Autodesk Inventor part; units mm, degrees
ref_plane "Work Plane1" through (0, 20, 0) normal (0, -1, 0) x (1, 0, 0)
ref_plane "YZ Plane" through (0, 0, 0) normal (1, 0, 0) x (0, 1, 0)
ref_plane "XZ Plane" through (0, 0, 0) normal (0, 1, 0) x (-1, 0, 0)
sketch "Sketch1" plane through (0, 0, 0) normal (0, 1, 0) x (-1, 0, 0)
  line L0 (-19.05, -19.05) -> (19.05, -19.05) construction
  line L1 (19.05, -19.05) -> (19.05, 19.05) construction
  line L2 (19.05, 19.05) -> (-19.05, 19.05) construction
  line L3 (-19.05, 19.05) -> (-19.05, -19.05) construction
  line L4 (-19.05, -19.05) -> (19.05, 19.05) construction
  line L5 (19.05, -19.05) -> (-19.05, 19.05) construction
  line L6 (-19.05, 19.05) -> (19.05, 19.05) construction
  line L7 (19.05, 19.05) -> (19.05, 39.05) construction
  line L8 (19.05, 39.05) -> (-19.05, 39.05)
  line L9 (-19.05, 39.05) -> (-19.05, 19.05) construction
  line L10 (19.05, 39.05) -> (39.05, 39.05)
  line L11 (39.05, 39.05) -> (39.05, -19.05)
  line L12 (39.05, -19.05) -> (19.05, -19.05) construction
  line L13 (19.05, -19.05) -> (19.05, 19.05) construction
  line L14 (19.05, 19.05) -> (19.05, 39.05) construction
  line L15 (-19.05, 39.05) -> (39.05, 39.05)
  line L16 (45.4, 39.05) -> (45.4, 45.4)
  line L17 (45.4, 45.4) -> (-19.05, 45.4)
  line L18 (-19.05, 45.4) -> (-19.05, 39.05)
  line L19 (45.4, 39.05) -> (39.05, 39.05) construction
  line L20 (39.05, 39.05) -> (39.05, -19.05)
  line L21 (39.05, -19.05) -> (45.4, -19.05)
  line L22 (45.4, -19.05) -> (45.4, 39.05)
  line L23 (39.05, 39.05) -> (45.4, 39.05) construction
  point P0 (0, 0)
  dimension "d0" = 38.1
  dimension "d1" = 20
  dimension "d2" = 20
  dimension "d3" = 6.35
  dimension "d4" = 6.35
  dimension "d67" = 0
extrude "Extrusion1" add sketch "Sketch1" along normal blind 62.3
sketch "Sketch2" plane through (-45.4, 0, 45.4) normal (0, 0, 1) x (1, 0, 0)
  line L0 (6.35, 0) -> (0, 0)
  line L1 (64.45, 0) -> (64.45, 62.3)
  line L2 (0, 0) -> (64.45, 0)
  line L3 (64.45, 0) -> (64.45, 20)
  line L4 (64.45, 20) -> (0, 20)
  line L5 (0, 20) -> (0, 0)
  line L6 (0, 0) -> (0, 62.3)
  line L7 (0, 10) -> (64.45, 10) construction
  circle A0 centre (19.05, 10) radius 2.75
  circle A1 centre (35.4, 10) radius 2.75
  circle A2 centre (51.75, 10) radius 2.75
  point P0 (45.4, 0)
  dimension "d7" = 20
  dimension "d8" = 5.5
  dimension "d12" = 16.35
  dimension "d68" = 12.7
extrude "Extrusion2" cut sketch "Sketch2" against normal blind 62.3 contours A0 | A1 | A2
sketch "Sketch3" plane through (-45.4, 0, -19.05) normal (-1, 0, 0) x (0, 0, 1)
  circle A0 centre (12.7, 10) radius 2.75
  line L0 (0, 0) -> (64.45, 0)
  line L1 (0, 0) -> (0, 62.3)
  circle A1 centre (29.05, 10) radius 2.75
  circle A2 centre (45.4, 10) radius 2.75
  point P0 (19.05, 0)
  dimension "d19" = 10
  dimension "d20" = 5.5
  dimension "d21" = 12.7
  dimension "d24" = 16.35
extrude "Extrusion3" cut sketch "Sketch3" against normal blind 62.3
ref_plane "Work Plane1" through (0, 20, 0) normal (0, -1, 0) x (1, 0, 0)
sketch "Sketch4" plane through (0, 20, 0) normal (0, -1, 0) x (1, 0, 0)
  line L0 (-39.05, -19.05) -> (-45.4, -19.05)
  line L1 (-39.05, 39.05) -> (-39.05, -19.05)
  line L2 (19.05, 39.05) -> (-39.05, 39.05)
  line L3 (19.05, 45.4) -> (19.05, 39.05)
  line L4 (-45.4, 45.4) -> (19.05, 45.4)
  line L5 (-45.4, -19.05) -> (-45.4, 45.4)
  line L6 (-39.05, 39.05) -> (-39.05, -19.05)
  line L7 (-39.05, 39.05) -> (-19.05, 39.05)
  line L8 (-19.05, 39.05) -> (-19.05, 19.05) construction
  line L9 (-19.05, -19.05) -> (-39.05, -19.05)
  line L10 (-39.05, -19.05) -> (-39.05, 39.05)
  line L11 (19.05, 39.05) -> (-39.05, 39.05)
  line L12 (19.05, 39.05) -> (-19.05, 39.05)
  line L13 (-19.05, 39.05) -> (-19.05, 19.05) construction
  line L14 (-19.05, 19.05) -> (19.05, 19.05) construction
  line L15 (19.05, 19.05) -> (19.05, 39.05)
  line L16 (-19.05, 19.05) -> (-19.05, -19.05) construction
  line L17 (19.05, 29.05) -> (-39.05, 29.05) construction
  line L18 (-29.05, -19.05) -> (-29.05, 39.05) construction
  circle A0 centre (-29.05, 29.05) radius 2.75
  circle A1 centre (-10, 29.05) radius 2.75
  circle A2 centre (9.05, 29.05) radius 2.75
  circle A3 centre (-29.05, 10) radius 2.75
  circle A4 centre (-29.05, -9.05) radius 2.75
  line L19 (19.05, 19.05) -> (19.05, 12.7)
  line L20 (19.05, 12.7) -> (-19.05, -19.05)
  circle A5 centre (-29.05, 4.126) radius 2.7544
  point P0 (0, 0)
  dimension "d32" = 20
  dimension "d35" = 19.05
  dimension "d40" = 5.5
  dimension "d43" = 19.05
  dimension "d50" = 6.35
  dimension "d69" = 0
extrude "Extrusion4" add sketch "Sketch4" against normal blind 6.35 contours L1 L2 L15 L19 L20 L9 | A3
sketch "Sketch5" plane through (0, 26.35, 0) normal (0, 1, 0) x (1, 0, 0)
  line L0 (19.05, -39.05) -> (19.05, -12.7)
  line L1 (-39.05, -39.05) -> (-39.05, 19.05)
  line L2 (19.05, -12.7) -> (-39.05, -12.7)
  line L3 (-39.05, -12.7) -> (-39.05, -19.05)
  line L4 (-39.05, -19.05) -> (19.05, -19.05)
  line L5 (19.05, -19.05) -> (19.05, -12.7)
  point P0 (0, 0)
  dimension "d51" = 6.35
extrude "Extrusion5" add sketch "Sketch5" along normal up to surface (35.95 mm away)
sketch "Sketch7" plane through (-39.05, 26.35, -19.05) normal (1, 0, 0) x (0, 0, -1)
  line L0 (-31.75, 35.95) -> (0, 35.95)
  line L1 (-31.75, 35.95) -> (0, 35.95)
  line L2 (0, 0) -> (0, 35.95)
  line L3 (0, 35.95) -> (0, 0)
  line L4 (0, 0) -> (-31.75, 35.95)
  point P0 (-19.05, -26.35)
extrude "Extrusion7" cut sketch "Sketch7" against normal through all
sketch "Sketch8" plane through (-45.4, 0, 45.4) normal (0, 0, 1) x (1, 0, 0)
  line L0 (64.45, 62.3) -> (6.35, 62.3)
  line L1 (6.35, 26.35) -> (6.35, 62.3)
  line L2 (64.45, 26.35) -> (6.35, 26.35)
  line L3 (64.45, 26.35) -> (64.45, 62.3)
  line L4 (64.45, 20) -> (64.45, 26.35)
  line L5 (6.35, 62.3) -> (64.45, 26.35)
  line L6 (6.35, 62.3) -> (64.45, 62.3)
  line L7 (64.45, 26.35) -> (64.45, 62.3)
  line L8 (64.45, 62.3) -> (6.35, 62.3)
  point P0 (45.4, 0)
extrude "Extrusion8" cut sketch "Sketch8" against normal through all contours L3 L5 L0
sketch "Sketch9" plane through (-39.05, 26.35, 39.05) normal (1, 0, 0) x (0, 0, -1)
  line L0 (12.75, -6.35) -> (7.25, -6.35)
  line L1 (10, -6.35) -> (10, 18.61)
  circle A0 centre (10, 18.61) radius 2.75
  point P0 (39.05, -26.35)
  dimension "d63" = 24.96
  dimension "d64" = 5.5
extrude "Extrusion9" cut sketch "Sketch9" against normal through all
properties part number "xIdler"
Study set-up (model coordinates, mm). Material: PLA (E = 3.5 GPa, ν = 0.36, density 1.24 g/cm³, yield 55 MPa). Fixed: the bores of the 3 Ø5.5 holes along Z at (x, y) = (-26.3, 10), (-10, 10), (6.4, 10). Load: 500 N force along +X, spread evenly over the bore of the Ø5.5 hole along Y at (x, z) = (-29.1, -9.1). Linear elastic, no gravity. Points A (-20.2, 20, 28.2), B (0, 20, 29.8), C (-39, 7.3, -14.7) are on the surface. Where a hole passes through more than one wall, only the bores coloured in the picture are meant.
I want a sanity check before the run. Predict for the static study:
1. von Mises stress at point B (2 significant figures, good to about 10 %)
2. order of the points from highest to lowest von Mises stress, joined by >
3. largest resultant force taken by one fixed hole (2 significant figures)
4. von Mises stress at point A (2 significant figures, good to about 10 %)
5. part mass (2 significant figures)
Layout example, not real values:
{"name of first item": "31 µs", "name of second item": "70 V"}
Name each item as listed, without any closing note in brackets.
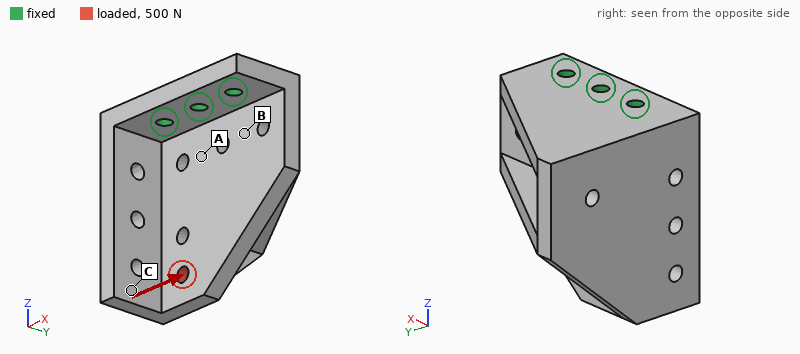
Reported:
{"von Mises stress at point B": "11 MPa", "order of the points from highest to lowest von Mises stress, joined by >": "B > A > C", "largest resultant force taken by one fixed hole": "700 N", "von Mises stress at point A": "6.2 MPa", "part mass": "75 g"}
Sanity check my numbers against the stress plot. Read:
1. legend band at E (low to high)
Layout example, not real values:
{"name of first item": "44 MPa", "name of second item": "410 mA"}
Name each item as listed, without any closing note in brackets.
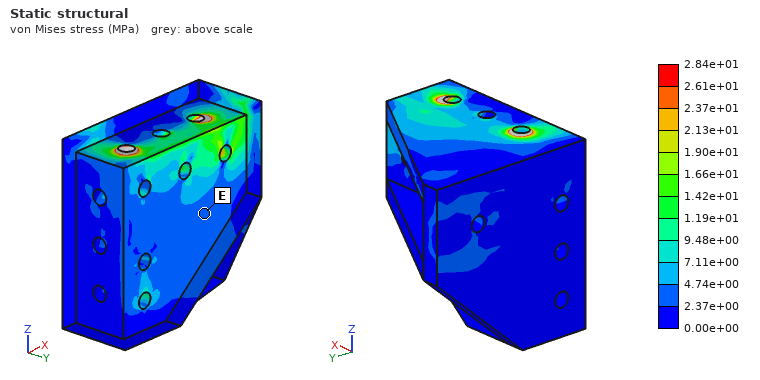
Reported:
{"legend band at E": "2.37e+00 to 4.74e+00 MPa"}
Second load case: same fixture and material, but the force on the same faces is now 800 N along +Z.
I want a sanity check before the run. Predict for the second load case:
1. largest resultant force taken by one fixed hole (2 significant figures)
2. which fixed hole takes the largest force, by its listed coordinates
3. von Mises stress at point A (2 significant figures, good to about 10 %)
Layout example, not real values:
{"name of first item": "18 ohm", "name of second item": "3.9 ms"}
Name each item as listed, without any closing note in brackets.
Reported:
{"largest resultant force taken by one fixed hole": "660 N", "which fixed hole takes the largest force, by its listed coordinates": "(-26.3, 10)", "von Mises stress at point A": "3.8 MPa"}
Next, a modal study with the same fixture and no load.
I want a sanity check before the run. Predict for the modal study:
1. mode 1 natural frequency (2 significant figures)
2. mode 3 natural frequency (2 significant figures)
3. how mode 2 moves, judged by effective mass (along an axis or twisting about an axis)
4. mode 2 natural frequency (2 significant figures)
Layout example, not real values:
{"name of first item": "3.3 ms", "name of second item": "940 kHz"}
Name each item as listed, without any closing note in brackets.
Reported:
{"mode 1 natural frequency": "370 Hz", "mode 3 natural frequency": "1300 Hz", "how mode 2 moves, judged by effective mass": "along X", "mode 2 natural frequency": "950 Hz"}
